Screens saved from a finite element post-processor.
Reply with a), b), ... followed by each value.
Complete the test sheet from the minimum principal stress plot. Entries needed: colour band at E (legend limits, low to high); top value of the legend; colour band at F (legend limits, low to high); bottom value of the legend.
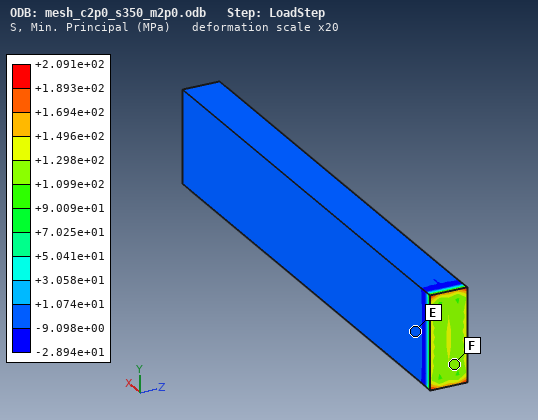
a) -9.098e+00 to +1.074e+01 MPa
b) +2.091e+02 MPa
c) +1.099e+02 to +1.298e+02 MPa
d) -2.894e+01 MPa
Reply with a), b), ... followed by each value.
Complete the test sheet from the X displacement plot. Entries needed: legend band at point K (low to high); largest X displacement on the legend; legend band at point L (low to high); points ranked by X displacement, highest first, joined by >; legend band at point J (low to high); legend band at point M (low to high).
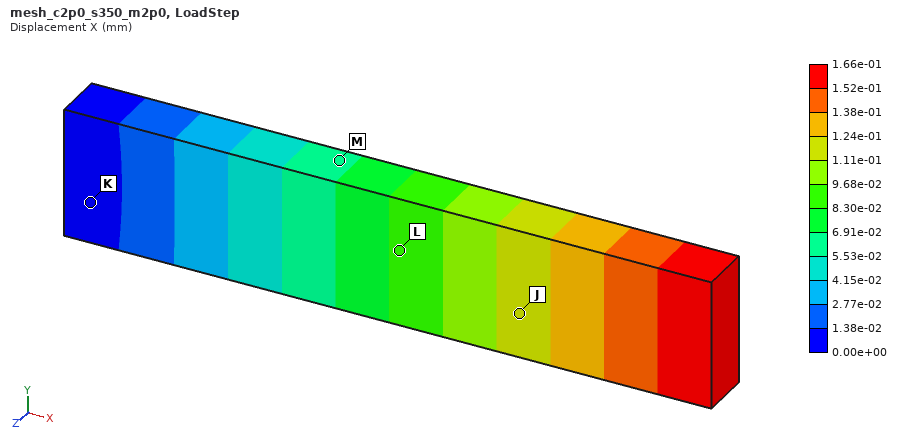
a) 0.00e+00 to 1.38e-02 mm
b) 1.66e-01 mm
c) 8.30e-02 to 9.68e-02 mm
d) J > L > M > K
e) 1.11e-01 to 1.24e-01 mm
f) 5.53e-02 to 6.91e-02 mm
